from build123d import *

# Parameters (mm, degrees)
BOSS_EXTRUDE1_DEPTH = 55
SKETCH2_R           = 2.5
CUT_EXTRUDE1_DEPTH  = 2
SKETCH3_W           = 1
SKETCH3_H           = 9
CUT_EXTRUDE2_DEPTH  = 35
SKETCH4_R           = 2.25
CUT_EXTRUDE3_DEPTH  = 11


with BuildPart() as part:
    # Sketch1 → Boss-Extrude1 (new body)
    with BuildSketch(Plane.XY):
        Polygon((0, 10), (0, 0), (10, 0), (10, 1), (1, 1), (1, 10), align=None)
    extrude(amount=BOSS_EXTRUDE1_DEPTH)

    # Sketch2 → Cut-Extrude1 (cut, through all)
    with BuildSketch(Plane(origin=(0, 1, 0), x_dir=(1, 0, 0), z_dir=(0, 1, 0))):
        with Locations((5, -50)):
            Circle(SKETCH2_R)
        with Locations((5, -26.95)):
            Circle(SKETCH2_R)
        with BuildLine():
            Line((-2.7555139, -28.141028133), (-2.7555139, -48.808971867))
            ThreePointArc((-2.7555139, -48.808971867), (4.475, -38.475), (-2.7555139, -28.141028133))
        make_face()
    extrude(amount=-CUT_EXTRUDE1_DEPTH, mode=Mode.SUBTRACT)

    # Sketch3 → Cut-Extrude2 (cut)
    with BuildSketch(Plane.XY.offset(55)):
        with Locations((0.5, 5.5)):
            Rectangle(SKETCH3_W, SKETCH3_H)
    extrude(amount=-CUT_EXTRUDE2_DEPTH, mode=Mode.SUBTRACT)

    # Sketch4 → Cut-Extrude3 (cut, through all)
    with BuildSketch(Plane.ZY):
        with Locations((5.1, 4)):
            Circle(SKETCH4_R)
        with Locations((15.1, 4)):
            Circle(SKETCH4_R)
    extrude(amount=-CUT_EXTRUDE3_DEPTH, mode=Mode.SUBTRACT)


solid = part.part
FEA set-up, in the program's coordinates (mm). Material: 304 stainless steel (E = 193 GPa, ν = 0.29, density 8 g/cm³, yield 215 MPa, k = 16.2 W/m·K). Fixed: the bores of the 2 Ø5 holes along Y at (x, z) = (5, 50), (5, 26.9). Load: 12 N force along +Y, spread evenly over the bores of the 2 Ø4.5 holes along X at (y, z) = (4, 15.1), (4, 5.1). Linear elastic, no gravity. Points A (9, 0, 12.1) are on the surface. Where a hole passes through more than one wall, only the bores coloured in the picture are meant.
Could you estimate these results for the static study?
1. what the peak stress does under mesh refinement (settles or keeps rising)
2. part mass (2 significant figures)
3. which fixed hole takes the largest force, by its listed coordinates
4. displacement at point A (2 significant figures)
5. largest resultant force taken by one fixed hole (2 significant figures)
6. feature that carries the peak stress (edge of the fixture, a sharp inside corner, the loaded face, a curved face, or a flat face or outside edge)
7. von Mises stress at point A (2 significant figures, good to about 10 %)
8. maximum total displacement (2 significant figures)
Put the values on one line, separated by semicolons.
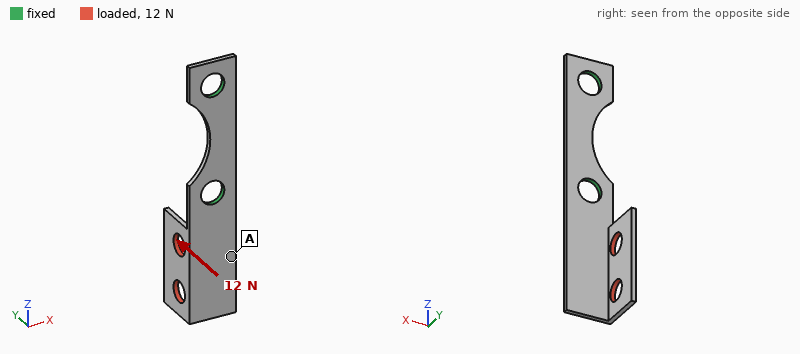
keeps rising; 4.8 g; (5, 26.9); 0.047 mm; 12 N; edge of the fixture; 15 MPa; 0.16 mm
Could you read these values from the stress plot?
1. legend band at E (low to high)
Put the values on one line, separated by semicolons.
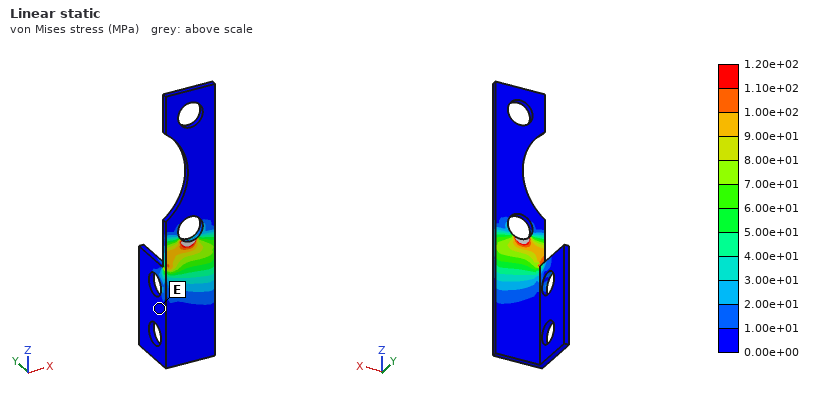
0.00e+00 to 1.00e+01 MPa
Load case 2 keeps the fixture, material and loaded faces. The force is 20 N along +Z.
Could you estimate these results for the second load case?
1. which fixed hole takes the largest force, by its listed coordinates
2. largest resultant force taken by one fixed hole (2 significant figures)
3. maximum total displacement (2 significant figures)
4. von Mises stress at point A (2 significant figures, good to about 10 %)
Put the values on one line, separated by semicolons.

(5, 26.9); 20 N; 79 µm; 8.1 MPa
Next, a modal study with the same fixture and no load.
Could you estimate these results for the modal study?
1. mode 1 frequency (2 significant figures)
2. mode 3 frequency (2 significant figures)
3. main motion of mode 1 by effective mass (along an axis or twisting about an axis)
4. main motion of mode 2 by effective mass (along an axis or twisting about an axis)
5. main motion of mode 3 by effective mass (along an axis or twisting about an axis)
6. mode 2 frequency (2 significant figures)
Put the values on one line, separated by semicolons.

1000 Hz; 7800 Hz; along Y; along X; along X; 2900 Hz
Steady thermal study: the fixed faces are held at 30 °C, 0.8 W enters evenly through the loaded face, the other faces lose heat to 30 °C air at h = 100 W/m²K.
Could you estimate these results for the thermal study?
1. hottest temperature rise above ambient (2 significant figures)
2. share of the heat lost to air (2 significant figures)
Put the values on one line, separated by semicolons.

15 K; 88 %
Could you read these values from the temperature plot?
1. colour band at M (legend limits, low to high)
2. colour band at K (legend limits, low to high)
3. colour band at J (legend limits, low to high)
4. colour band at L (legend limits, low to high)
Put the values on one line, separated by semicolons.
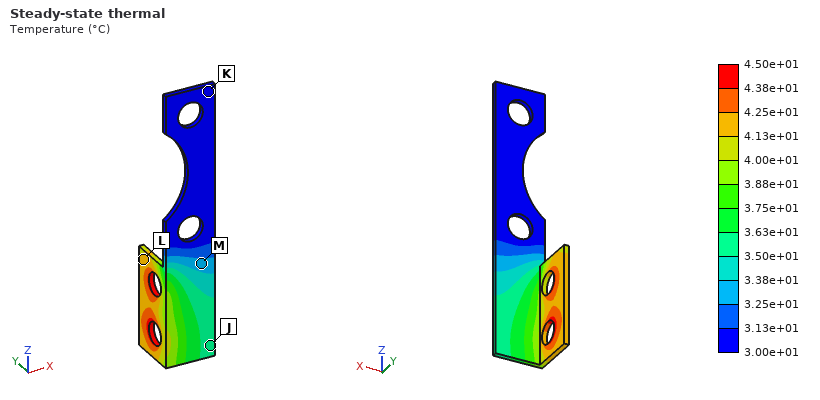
3.25e+01 to 3.38e+01 °C; 3.00e+01 to 3.13e+01 °C; 3.50e+01 to 3.63e+01 °C; 4.13e+01 to 4.25e+01 °C
